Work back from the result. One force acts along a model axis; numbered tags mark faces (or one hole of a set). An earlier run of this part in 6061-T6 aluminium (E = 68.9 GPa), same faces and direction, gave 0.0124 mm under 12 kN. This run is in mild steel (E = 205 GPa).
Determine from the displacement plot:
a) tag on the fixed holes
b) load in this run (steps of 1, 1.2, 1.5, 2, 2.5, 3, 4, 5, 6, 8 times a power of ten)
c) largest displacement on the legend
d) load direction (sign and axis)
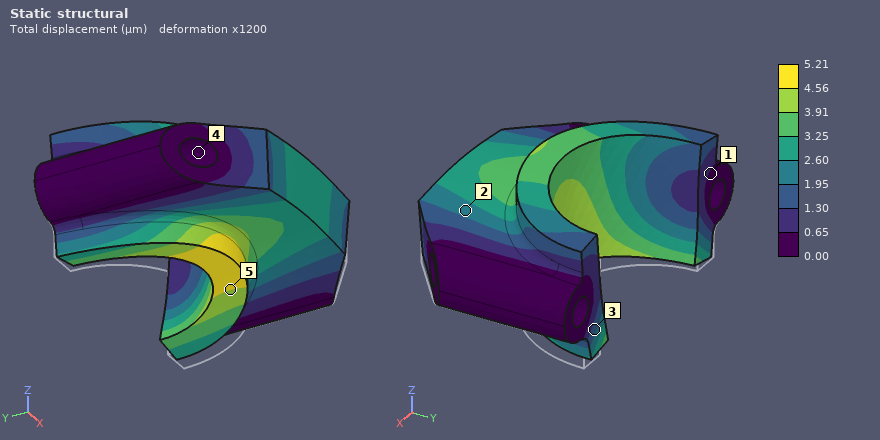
4
15 kN
5.21 µm
+Z
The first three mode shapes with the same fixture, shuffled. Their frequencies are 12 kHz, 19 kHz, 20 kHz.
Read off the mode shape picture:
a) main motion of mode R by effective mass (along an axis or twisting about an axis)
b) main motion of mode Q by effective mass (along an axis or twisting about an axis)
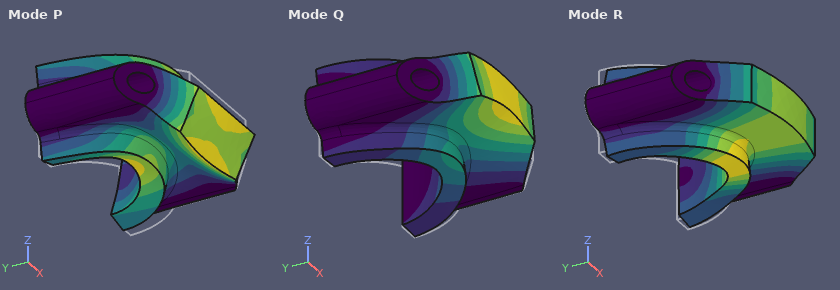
along Y
along Z
